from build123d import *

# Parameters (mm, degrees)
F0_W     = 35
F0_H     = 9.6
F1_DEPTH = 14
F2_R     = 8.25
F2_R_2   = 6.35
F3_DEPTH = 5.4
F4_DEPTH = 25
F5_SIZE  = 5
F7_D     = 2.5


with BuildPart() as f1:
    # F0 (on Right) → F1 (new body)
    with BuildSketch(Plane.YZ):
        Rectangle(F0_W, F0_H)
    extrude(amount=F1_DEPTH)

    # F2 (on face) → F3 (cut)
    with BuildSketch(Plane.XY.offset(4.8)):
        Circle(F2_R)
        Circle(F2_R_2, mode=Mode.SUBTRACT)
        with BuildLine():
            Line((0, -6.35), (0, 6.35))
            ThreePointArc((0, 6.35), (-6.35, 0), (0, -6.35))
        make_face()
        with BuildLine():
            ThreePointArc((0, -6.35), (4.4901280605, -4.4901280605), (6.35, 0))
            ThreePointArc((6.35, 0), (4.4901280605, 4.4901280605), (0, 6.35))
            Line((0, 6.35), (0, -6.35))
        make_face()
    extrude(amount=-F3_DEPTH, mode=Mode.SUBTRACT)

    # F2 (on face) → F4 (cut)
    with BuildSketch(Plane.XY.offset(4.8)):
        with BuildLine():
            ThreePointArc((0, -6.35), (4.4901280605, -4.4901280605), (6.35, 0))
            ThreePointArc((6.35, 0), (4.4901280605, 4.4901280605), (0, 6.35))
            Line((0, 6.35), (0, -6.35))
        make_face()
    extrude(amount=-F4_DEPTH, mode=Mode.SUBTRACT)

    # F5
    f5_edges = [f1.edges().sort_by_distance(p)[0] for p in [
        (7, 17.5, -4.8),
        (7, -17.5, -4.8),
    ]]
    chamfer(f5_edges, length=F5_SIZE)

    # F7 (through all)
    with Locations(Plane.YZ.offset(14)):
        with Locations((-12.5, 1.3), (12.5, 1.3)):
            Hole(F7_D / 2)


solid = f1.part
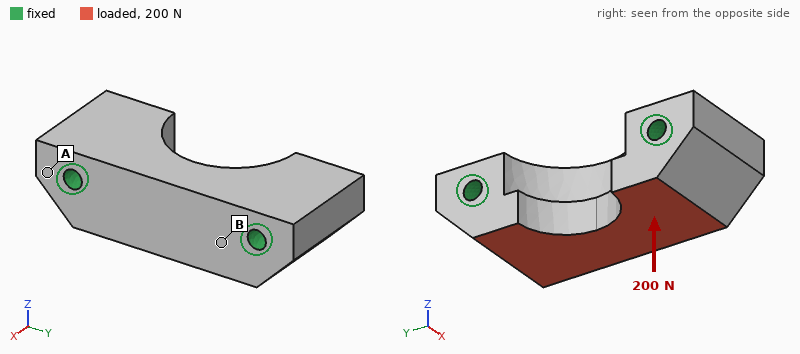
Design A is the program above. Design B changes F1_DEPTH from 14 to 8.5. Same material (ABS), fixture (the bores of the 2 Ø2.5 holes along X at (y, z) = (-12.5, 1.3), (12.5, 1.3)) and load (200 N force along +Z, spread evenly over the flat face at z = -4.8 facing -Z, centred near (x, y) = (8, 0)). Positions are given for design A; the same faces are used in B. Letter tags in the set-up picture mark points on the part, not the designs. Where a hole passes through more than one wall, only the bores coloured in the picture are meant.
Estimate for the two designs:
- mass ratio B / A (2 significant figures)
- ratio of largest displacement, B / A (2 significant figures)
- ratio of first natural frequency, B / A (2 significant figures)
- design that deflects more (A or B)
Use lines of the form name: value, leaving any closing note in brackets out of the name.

mass ratio B / A: 0.51
ratio of largest displacement, B / A: 2.2
ratio of first natural frequency, B / A: 1.1
design that deflects more: B
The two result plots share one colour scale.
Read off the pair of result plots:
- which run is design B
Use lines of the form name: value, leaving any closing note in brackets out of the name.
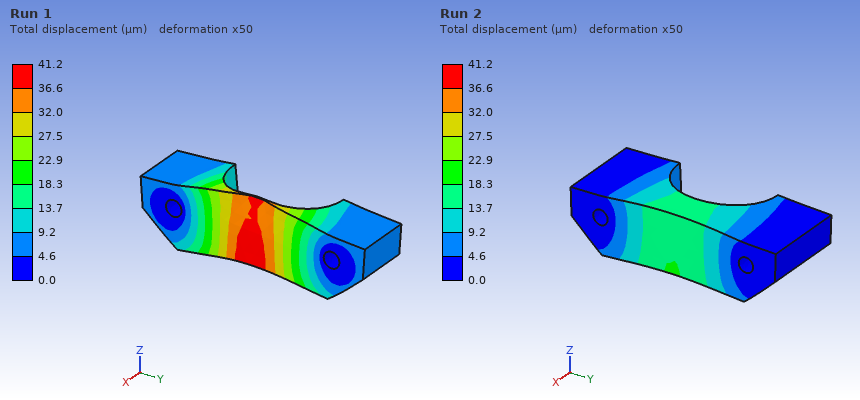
which run is design B: Run 1
